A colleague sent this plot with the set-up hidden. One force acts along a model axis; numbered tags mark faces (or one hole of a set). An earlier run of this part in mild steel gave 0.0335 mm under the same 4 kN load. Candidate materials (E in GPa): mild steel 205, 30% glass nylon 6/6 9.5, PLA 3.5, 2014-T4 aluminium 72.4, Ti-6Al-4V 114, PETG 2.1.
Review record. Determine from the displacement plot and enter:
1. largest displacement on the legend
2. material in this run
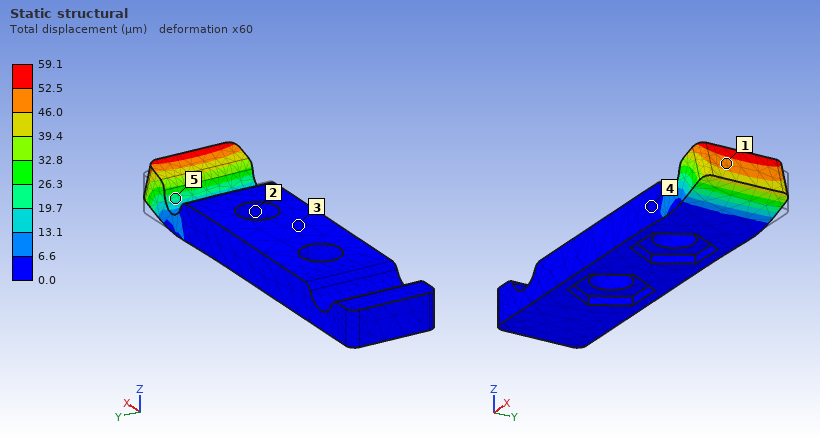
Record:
59.1 µm
Ti-6Al-4V
